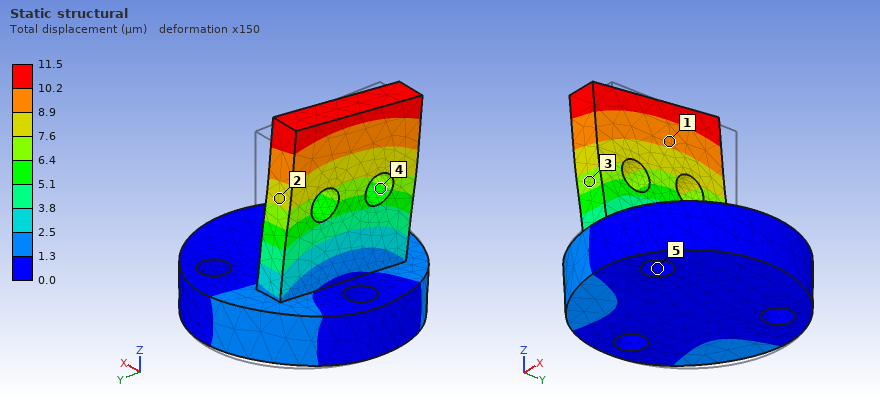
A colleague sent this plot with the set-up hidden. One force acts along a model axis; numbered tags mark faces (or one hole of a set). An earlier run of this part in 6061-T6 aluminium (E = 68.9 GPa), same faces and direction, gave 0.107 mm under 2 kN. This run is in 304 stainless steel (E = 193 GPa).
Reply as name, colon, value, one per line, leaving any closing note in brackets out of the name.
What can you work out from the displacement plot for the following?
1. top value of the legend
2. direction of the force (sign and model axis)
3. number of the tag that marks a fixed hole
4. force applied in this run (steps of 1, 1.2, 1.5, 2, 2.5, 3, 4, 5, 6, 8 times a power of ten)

top value of the legend: 11.5 µm
direction of the force: -Y
number of the tag that marks a fixed hole: 5
force applied in this run: 600 N
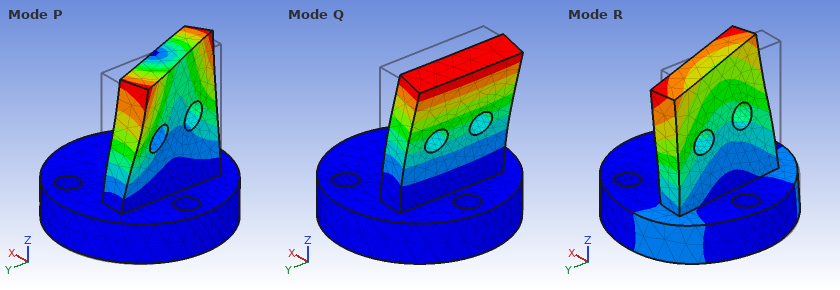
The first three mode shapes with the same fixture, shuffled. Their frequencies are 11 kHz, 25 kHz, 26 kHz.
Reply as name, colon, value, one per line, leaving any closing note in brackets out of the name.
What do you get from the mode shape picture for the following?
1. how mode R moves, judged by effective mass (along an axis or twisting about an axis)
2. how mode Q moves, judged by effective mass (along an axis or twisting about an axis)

how mode R moves, judged by effective mass: along Y
how mode Q moves, judged by effective mass: along X
